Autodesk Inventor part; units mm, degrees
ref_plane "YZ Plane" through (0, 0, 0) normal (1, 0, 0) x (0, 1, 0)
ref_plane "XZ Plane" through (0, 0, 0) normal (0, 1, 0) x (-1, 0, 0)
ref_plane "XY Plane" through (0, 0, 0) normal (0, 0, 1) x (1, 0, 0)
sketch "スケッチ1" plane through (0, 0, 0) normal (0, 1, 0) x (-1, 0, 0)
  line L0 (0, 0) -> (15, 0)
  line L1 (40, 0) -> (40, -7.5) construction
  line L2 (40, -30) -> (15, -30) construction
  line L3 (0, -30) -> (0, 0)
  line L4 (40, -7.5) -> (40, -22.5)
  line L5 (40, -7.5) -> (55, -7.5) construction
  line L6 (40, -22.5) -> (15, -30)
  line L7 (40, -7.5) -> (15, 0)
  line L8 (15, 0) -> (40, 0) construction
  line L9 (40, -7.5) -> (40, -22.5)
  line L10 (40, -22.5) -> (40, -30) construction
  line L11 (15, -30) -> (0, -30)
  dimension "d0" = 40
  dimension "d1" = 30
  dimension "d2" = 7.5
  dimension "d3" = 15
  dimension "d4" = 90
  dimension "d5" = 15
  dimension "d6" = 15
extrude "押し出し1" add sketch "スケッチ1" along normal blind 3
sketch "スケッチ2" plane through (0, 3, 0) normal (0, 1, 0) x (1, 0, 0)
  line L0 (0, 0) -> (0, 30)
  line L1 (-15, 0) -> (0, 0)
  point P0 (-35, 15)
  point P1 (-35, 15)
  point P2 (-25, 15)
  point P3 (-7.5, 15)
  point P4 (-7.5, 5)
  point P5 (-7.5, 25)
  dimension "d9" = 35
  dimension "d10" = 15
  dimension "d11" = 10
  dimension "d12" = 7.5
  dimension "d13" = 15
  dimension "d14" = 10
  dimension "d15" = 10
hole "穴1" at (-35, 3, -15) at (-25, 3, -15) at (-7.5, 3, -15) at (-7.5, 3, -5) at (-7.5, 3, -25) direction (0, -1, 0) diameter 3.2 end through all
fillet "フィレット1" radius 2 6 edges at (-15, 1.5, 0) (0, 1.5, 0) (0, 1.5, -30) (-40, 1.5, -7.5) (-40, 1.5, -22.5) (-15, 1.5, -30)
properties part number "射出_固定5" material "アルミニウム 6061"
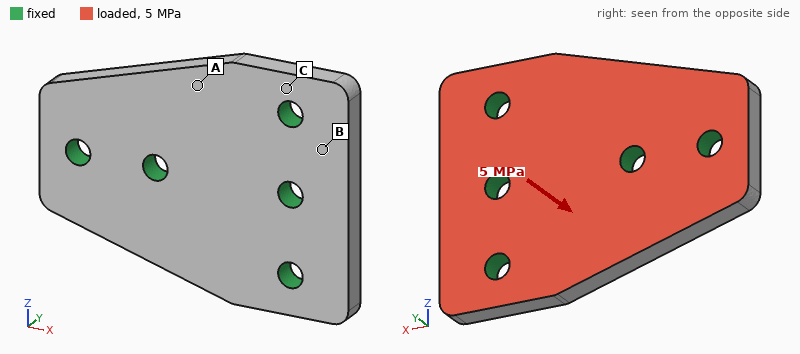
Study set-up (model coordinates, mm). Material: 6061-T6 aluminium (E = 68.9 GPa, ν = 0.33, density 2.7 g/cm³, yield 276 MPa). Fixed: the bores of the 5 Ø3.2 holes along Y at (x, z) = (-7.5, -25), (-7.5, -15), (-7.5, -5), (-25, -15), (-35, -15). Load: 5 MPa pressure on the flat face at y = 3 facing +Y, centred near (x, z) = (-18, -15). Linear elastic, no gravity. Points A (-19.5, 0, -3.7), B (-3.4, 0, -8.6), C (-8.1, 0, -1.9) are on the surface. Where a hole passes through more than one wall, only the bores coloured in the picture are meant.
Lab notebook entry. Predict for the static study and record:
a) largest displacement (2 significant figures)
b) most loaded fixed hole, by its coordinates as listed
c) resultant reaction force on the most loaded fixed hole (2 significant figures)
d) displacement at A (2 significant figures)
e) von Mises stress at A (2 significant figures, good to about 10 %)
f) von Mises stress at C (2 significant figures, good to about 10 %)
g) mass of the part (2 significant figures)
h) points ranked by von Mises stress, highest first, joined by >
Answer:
46 µm
(-25, -15)
1.4 kN
35 µm
55 MPa
74 MPa
7.9 g
C > A > B
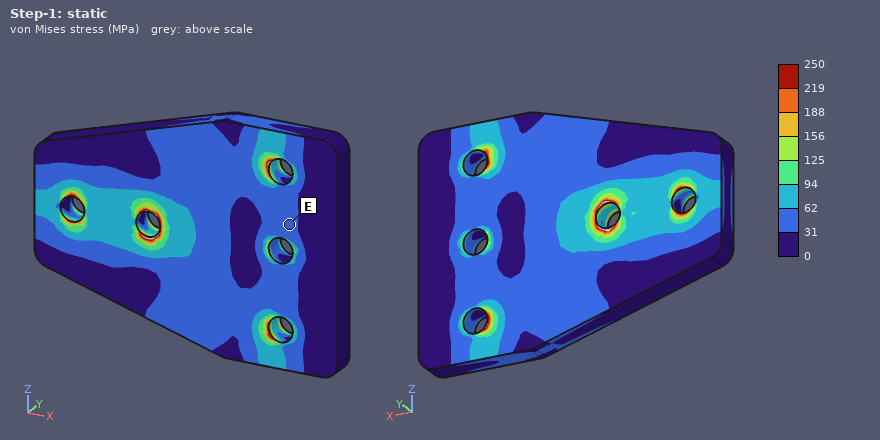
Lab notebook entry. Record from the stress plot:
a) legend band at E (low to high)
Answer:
31 to 62 MPa
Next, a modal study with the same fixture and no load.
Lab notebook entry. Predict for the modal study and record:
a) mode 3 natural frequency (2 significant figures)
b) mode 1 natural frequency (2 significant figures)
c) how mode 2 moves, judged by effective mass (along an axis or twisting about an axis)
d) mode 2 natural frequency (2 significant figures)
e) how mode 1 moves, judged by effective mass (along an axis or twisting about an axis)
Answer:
38 kHz
23 kHz
along Y
25 kHz
twisting about X
